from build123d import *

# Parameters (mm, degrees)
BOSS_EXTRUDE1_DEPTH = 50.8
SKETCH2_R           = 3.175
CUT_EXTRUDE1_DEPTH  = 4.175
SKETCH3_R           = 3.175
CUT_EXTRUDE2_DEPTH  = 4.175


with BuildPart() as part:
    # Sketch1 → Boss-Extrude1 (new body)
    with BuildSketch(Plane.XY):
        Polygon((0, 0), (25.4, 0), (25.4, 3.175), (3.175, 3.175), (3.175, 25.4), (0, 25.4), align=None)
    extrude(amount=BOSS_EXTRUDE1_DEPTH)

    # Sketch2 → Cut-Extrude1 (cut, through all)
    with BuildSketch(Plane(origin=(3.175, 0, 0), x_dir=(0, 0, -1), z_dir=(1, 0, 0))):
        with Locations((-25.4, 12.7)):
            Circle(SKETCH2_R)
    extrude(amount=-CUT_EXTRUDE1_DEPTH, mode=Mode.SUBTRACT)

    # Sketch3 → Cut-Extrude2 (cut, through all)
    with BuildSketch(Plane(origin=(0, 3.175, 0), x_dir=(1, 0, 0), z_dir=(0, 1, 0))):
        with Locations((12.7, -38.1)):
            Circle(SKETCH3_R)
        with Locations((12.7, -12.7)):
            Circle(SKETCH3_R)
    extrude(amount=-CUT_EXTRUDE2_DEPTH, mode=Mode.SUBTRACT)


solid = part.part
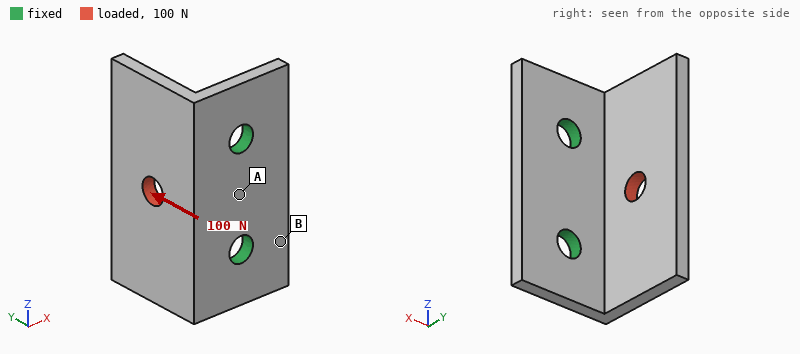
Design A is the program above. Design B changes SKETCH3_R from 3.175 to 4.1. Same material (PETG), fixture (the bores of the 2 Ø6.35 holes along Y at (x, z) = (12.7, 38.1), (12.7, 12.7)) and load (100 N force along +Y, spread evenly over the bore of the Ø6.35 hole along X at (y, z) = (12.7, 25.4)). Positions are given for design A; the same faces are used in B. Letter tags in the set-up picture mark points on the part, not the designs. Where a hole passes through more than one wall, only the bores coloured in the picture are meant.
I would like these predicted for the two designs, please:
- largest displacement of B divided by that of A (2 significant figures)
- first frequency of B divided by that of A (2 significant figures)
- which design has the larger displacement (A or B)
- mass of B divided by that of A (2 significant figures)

0.78
1.1
A
0.98
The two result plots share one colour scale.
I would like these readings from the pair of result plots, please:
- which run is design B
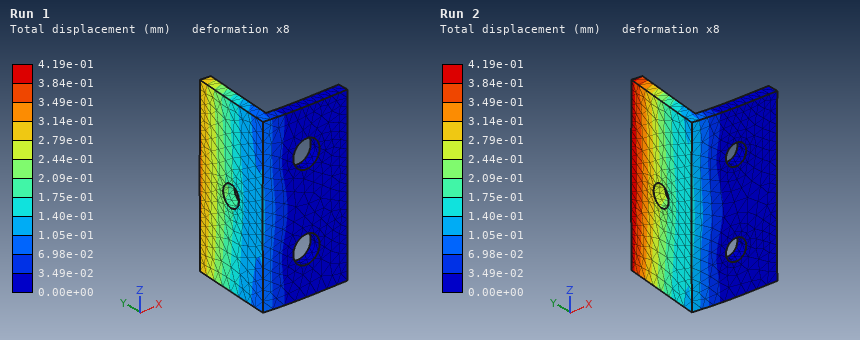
Run 1
